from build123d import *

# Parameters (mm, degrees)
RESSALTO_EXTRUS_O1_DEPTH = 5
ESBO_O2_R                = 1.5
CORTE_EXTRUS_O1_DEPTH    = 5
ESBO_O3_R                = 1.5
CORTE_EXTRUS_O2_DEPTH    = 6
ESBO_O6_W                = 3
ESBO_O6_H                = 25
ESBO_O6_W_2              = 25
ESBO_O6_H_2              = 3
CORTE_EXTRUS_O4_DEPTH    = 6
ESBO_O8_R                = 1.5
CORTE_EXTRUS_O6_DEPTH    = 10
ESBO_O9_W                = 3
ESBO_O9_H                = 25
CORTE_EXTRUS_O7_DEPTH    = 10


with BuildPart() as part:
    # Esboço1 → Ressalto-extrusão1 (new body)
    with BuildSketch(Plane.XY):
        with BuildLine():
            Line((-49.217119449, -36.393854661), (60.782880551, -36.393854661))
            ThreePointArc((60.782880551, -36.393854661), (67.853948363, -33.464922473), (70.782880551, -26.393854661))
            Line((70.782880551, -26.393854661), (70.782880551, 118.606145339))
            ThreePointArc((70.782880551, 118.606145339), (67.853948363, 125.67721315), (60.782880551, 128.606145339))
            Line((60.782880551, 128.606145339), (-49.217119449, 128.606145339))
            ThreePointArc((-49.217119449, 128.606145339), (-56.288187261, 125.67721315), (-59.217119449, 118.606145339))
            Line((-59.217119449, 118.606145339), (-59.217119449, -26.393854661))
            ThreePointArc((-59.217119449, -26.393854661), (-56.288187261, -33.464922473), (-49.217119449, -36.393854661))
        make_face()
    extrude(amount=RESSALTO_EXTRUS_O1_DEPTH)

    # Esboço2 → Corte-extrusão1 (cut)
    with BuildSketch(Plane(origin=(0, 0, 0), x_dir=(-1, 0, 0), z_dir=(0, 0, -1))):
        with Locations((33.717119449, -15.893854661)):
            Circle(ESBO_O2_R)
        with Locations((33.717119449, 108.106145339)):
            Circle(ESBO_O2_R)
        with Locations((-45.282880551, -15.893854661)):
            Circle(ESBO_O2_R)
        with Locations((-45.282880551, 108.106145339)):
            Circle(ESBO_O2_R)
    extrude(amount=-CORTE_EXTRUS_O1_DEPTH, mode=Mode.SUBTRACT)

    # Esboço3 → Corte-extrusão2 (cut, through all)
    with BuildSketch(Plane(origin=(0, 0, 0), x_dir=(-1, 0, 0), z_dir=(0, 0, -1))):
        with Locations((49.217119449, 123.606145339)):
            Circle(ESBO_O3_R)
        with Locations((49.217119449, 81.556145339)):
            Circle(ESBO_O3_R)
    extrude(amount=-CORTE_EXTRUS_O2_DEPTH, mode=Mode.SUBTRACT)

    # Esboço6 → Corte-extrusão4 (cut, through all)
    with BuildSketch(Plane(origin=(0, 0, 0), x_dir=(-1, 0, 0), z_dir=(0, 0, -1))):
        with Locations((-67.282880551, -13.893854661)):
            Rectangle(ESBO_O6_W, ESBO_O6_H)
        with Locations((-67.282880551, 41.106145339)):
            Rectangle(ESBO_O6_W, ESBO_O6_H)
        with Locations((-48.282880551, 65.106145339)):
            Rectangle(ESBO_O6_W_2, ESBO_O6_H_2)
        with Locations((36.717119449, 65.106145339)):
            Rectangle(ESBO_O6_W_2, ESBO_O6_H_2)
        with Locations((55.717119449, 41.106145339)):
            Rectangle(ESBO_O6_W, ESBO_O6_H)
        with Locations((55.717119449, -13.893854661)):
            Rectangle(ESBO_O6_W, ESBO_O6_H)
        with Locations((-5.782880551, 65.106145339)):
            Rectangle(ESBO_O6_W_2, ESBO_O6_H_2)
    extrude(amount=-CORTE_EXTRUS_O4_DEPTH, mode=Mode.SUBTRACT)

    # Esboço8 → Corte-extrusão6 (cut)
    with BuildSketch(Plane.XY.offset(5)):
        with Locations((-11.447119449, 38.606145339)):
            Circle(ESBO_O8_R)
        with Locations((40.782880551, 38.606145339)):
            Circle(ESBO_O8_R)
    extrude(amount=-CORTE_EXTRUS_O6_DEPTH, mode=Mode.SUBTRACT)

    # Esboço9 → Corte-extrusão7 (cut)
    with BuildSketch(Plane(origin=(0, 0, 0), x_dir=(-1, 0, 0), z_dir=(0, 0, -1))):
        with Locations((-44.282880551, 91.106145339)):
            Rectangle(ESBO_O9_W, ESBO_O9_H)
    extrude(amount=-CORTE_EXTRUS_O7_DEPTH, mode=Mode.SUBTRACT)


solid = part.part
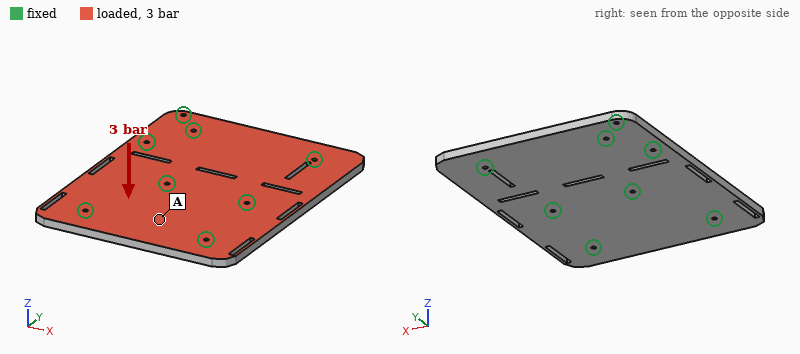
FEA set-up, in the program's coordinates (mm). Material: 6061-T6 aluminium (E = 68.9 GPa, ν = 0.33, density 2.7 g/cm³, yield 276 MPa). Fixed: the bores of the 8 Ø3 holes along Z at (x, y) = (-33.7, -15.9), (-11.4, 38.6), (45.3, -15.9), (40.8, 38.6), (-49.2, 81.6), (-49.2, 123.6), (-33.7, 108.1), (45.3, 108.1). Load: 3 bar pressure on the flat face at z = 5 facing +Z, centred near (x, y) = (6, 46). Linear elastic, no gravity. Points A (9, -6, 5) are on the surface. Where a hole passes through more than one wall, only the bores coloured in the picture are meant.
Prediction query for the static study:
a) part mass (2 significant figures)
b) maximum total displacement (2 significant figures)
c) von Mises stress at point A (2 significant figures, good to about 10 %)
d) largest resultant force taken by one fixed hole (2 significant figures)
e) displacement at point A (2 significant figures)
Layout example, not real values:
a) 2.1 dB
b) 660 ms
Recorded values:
a) 280 g
b) 83 µm
c) 12 MPa
d) 1.1 kN
e) 38 µm
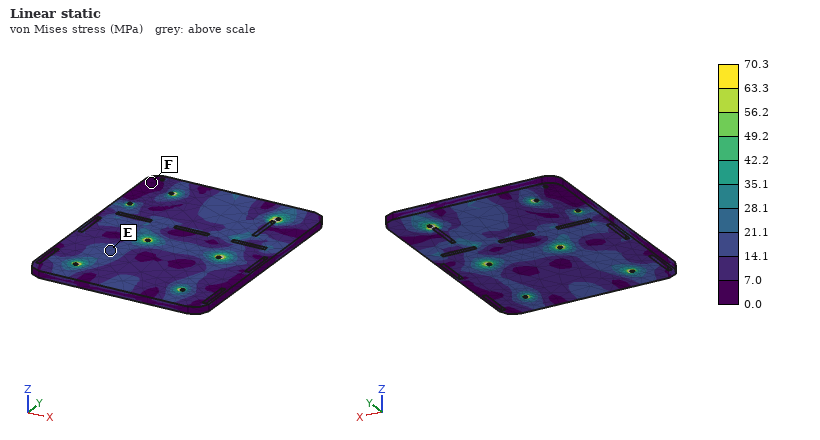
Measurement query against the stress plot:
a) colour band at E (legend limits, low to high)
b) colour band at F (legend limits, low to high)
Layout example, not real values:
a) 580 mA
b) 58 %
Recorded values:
a) 14.1 to 21.1 MPa
b) 0.0 to 7.0 MPa
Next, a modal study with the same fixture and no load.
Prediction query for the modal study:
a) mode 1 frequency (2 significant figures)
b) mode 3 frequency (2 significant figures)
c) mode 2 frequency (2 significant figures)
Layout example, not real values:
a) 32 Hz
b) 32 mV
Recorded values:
a) 2900 Hz
b) 3300 Hz
c) 3200 Hz
